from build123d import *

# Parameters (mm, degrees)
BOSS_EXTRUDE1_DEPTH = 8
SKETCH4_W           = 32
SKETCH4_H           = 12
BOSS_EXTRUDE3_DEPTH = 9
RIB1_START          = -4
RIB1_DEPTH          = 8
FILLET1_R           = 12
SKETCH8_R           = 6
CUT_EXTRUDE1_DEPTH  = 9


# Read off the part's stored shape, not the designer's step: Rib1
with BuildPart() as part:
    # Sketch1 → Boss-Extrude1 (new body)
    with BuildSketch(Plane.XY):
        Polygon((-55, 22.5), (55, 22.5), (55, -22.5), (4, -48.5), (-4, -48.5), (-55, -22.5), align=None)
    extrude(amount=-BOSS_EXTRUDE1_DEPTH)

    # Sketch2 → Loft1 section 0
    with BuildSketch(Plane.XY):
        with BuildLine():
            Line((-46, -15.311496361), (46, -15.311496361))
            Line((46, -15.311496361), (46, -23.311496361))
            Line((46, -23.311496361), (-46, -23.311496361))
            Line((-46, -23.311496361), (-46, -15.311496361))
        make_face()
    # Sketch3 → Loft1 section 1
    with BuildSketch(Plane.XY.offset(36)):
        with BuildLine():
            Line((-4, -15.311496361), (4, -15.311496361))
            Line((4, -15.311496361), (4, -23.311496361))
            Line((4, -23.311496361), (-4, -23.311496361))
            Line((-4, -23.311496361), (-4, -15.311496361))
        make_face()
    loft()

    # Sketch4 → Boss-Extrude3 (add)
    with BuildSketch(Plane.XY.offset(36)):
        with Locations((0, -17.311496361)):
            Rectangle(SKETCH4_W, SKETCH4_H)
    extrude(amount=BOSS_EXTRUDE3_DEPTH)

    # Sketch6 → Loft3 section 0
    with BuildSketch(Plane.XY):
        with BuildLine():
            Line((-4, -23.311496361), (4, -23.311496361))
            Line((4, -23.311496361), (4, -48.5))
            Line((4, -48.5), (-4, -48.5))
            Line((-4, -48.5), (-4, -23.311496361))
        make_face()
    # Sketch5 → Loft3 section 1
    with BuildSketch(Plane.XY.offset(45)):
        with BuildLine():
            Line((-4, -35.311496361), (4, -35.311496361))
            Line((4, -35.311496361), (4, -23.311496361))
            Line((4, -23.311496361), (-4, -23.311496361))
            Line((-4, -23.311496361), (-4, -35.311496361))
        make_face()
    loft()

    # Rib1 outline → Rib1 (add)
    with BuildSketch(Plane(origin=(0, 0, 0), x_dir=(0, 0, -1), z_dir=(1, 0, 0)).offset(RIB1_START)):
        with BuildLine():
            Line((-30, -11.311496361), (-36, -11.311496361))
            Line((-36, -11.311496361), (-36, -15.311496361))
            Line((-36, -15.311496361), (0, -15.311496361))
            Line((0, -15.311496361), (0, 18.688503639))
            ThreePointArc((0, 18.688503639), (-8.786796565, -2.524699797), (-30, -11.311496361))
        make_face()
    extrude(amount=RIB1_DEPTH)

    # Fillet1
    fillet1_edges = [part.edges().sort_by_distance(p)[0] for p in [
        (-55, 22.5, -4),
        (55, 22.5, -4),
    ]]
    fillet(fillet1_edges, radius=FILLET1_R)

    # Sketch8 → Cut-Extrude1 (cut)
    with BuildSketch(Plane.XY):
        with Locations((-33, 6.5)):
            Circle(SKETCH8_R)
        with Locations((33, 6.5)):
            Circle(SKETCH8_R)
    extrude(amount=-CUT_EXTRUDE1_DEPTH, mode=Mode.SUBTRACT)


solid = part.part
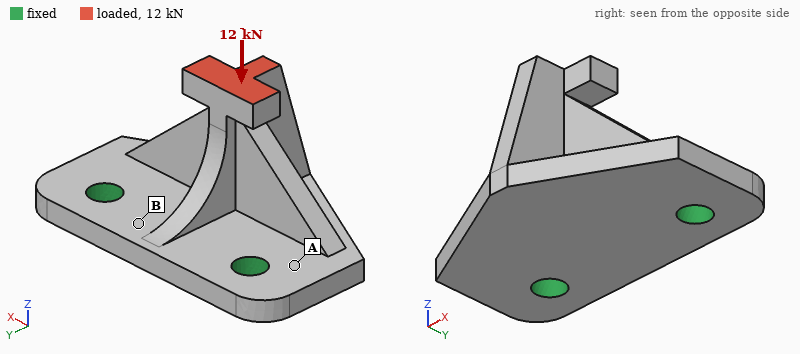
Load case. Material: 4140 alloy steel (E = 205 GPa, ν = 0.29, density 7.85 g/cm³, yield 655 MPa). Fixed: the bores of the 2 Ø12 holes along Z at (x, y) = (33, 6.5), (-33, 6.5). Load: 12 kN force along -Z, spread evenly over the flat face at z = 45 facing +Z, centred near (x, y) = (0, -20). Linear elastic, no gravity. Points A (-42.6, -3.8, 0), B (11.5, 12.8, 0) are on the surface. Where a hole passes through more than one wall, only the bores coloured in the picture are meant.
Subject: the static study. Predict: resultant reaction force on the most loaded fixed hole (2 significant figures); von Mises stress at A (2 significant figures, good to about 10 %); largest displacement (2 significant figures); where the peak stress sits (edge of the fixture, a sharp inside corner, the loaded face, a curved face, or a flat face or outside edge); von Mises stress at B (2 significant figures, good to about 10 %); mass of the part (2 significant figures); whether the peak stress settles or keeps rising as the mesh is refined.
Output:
6.1 kN
140 MPa
0.21 mm
edge of the fixture
66 MPa
600 g
keeps rising
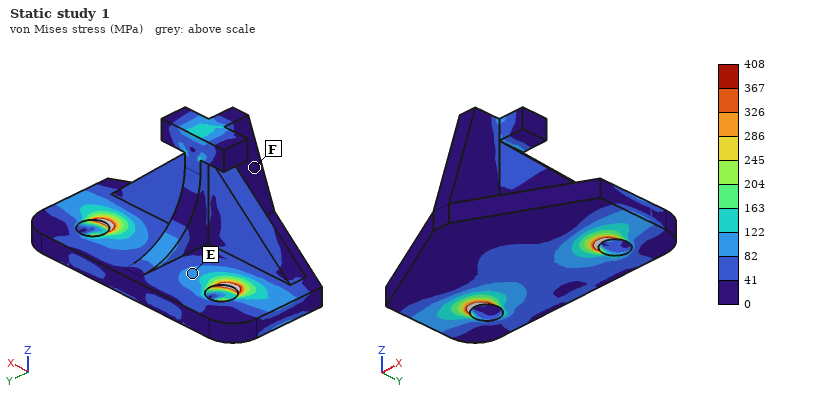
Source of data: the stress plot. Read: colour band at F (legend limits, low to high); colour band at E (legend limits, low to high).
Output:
0 to 41 MPa
82 to 122 MPa
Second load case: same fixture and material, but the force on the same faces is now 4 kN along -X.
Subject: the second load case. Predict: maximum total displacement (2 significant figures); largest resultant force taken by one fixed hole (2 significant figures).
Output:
76 µm
3.7 kN
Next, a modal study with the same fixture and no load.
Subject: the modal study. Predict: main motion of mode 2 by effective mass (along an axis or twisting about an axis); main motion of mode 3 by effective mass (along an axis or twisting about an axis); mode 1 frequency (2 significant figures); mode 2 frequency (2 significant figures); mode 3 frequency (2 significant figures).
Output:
along X
along Z
2100 Hz
4900 Hz
6300 Hz
